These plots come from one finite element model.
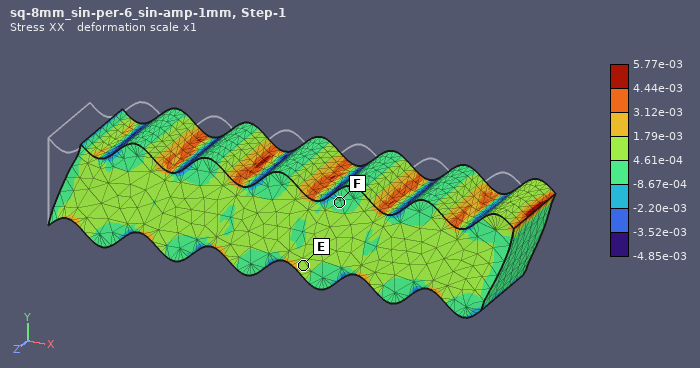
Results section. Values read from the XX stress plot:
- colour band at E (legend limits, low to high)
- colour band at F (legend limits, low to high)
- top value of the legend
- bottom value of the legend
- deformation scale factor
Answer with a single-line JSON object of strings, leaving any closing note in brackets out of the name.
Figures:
{"colour band at E": "4.61e-04 to 1.79e-03", "colour band at F": "-8.67e-04 to 4.61e-04", "top value of the legend": "5.77e-03", "bottom value of the legend": "-4.85e-03", "deformation scale factor": "1"}
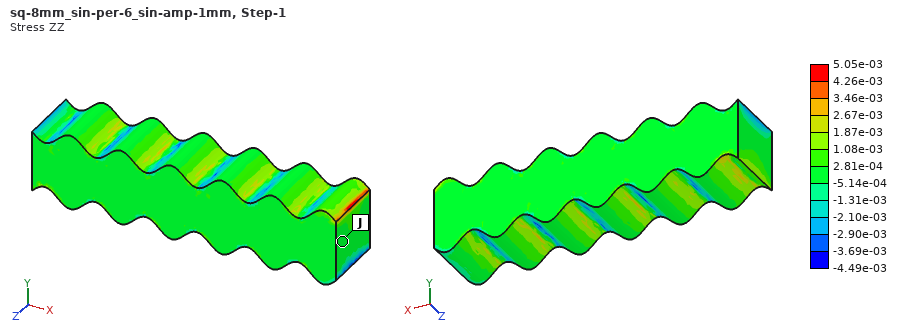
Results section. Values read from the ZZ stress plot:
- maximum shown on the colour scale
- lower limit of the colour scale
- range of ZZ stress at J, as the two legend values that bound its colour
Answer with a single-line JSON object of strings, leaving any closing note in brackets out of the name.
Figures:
{"maximum shown on the colour scale": "5.05e-03", "lower limit of the colour scale": "-4.49e-03", "range of ZZ stress at J, as the two legend values that bound its colour": "-5.14e-04 to 2.81e-04"}
